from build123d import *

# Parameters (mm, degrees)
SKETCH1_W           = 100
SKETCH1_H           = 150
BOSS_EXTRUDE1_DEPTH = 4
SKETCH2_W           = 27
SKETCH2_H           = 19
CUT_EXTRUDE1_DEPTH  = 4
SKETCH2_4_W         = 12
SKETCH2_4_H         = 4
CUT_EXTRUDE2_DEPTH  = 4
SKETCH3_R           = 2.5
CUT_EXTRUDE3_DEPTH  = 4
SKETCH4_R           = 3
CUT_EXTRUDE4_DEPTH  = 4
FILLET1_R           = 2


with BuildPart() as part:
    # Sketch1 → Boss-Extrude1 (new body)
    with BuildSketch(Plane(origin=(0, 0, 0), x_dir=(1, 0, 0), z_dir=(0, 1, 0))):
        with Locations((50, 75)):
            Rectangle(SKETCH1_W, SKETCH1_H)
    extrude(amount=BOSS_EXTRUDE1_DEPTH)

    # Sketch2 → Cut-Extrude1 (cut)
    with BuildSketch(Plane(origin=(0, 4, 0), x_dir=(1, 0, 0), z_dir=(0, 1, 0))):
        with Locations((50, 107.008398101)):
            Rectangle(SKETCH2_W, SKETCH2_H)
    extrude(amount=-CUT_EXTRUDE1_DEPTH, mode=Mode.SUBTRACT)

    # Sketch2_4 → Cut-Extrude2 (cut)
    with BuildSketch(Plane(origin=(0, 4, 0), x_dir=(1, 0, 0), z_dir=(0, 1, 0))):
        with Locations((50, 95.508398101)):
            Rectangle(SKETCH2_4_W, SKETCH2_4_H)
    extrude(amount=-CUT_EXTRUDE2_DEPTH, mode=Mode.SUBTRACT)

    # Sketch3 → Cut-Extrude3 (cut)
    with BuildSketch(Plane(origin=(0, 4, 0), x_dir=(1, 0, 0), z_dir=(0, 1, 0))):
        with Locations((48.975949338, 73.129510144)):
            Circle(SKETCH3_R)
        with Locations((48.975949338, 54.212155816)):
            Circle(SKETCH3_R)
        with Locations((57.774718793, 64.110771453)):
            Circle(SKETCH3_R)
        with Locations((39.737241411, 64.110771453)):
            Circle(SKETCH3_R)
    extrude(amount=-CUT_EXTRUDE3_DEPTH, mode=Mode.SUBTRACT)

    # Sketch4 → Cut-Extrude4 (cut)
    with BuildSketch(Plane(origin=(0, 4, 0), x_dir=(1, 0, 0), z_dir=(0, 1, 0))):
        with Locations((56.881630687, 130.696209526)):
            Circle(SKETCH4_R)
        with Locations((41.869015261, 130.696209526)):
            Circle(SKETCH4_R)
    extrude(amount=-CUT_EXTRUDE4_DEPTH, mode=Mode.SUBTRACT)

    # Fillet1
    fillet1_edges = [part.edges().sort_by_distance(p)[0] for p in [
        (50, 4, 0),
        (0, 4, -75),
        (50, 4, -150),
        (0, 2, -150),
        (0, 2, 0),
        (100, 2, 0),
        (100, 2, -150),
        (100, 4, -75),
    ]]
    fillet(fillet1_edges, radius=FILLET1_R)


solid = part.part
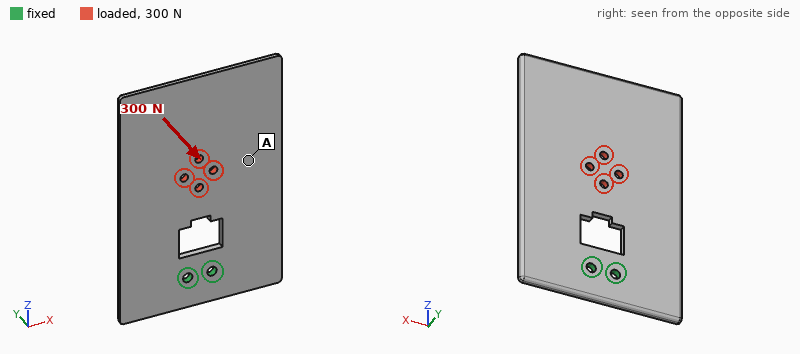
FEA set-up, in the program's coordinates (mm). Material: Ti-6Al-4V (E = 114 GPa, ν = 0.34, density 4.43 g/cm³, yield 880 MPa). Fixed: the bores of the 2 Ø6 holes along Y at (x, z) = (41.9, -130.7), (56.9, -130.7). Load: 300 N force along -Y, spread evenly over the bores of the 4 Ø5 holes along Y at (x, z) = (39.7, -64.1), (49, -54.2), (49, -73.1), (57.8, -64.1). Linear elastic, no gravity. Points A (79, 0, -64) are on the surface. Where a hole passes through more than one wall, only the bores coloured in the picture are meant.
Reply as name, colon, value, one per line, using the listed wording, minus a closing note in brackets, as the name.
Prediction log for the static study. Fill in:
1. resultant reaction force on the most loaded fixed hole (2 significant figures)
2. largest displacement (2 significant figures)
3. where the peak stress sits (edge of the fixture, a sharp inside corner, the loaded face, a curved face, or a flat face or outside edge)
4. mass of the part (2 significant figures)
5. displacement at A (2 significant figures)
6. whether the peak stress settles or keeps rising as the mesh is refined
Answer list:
resultant reaction force on the most loaded fixed hole: 160 N
largest displacement: 2.0 mm
where the peak stress sits: edge of the fixture
mass of the part: 250 g
displacement at A: 0.83 mm
whether the peak stress settles or keeps rising as the mesh is refined: keeps rising
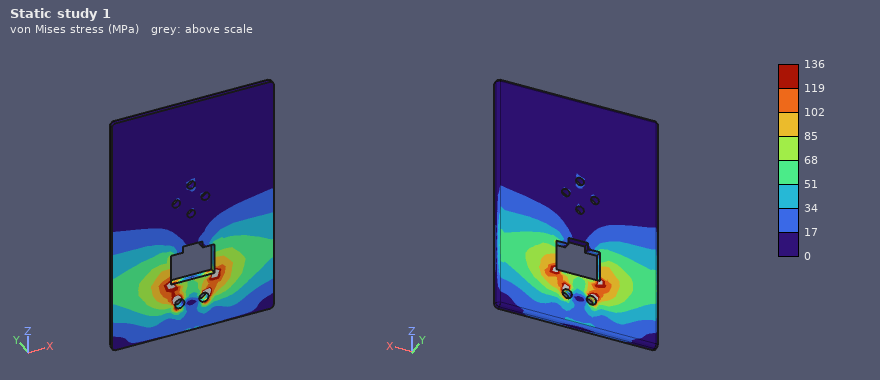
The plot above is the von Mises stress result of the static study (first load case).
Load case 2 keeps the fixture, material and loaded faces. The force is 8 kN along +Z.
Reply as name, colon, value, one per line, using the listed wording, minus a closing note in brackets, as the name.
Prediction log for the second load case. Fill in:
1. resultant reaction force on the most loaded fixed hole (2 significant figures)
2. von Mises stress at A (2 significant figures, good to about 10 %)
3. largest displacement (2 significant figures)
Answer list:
resultant reaction force on the most loaded fixed hole: 4.2 kN
von Mises stress at A: 15 MPa
largest displacement: 43 µm
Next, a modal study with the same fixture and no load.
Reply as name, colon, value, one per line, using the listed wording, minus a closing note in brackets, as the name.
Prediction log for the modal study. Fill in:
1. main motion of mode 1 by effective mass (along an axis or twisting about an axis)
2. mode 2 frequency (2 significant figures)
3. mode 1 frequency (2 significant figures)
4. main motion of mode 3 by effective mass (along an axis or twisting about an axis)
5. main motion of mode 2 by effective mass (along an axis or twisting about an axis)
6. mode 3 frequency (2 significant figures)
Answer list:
main motion of mode 1 by effective mass: along Y
mode 2 frequency: 450 Hz
mode 1 frequency: 160 Hz
main motion of mode 3 by effective mass: along Y
main motion of mode 2 by effective mass: twisting about Z
mode 3 frequency: 1000 Hz
